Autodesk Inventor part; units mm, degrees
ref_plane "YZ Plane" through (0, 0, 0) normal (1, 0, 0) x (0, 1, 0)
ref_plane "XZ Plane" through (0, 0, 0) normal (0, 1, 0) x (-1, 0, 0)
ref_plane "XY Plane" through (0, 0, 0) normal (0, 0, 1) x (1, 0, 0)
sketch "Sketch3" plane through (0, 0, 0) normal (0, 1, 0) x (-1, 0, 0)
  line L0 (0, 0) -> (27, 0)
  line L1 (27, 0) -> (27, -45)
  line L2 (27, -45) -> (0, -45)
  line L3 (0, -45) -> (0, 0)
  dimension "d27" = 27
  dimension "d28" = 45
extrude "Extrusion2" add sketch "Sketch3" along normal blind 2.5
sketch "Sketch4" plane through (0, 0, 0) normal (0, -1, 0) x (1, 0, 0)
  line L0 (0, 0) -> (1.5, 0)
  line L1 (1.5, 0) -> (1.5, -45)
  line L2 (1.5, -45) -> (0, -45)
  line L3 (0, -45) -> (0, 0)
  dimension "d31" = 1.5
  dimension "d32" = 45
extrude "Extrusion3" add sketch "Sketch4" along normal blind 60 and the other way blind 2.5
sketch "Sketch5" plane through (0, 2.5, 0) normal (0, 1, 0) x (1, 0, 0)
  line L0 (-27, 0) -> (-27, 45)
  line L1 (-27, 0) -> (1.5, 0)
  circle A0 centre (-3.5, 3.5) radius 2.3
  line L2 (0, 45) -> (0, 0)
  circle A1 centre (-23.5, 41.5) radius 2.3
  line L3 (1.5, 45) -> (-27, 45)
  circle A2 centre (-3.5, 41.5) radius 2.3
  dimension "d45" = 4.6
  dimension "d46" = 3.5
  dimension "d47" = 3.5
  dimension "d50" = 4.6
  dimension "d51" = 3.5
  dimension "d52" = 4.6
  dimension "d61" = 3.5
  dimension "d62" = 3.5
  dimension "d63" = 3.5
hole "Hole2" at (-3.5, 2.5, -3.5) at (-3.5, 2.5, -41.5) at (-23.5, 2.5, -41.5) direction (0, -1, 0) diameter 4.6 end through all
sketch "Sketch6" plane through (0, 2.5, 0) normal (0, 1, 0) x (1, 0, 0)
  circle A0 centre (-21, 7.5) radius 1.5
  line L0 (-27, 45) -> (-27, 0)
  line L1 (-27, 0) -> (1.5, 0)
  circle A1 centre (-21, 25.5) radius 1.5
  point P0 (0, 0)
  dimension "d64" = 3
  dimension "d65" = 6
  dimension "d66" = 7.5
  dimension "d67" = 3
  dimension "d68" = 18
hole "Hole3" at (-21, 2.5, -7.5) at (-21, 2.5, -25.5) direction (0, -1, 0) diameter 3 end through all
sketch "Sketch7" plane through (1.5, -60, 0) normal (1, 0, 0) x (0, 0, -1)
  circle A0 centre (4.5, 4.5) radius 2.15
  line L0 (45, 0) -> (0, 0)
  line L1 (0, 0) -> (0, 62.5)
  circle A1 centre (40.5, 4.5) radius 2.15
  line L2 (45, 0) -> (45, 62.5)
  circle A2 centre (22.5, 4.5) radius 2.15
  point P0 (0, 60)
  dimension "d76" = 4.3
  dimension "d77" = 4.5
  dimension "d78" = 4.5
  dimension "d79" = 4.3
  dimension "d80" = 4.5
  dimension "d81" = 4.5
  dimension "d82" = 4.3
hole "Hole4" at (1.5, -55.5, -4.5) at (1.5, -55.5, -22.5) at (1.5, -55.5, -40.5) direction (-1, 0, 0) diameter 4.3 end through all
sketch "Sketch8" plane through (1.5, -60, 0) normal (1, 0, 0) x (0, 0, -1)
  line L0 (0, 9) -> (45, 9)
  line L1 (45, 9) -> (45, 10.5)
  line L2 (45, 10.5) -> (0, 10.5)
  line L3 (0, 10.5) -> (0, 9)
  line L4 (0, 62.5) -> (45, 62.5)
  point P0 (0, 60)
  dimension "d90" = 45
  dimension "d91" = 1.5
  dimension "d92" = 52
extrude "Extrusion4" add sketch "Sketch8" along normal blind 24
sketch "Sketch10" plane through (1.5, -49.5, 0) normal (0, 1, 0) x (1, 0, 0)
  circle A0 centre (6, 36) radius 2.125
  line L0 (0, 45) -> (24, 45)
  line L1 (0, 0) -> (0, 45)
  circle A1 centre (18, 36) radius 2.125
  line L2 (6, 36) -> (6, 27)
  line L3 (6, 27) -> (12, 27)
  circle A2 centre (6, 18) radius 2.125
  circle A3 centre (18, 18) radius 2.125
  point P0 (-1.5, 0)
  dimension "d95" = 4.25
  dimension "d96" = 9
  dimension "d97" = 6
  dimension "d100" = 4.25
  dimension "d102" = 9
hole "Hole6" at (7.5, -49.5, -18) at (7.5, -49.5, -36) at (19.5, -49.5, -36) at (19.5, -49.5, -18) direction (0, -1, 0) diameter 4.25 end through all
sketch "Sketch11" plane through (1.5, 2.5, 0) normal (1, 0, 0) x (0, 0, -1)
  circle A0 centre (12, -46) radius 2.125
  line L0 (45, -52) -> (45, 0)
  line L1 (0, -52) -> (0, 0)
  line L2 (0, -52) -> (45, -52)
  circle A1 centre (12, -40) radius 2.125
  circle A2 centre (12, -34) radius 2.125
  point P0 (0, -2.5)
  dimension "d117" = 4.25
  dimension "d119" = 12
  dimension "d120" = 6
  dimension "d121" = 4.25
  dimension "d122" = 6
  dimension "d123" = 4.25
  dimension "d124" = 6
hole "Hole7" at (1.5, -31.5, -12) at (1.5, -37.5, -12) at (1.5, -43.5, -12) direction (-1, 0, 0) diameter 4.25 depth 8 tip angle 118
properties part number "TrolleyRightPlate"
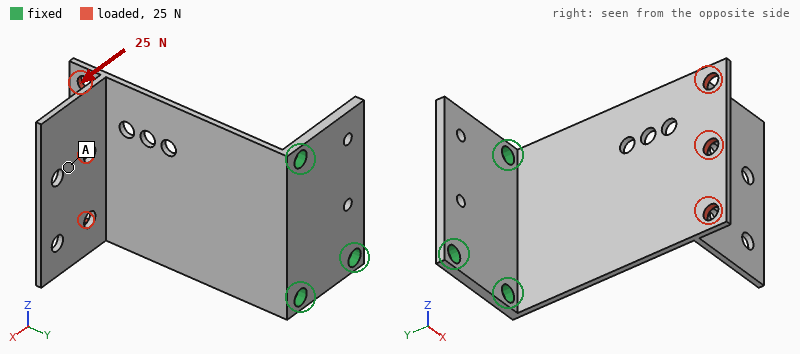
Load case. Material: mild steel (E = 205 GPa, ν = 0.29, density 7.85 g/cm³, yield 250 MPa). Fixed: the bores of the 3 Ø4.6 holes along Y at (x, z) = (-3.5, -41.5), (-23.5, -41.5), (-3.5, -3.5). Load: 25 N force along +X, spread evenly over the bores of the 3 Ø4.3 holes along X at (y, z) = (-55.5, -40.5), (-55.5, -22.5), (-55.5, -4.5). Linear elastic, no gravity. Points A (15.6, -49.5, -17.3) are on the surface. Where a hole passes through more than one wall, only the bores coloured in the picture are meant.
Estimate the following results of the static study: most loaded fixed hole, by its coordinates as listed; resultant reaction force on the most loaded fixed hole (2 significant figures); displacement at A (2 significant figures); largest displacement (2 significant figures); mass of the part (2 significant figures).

(-3.5, -41.5)
23 N
0.53 mm
0.64 mm
67 g
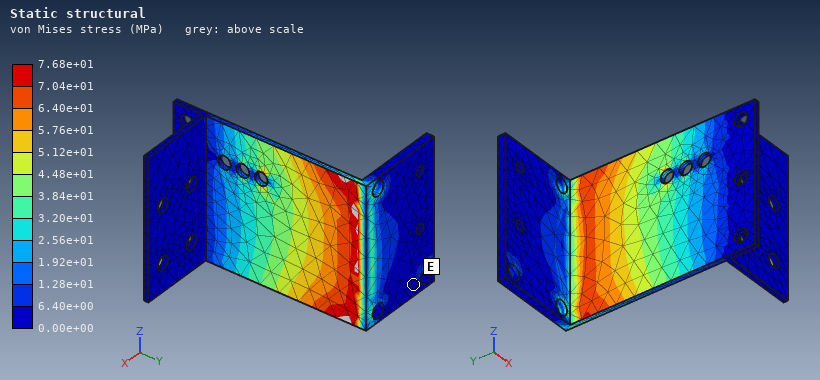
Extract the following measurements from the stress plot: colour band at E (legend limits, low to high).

0.00e+00 to 6.40e+00 MPa
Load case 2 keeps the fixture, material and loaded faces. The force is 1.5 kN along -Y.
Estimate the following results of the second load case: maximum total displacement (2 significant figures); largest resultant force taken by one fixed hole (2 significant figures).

58 µm
800 N
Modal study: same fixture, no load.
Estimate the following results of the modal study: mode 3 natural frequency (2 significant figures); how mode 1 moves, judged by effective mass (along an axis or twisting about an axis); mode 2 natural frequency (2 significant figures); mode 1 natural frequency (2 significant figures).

1100 Hz
along X
640 Hz
240 Hz
